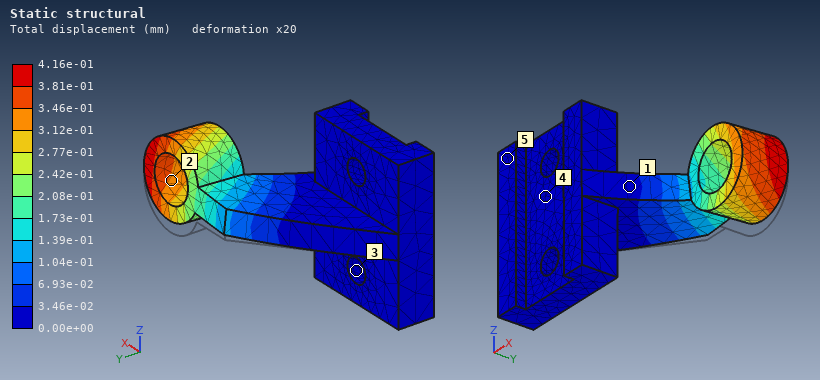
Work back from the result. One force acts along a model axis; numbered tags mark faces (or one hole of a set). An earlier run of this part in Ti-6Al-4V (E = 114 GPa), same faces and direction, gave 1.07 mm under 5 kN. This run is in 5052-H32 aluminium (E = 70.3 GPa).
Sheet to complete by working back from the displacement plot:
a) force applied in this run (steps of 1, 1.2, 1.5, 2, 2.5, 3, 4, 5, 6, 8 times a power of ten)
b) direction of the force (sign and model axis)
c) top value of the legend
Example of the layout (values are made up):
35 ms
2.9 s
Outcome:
1.2 kN
+Z
4.16e-01 mm
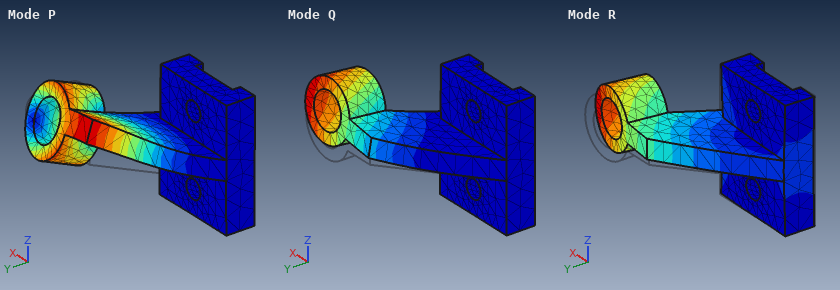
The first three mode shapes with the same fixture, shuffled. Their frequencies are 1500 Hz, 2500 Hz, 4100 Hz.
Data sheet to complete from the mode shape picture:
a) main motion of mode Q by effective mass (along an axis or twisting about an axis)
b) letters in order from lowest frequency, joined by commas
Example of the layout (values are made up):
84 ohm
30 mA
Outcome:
along Z
Q, R, P
